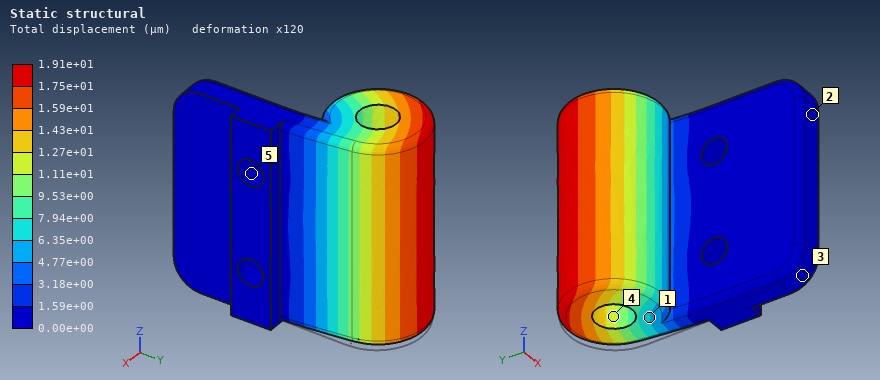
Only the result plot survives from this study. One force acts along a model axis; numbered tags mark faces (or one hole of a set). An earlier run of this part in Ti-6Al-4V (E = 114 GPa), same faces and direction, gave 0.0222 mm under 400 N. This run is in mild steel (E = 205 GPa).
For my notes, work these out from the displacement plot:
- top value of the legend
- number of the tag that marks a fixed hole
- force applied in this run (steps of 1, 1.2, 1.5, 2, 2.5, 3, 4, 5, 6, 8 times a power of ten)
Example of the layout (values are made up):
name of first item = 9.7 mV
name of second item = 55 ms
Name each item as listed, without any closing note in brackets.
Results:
top value of the legend = 1.91e+01 µm
number of the tag that marks a fixed hole = 5
force applied in this run = 600 N
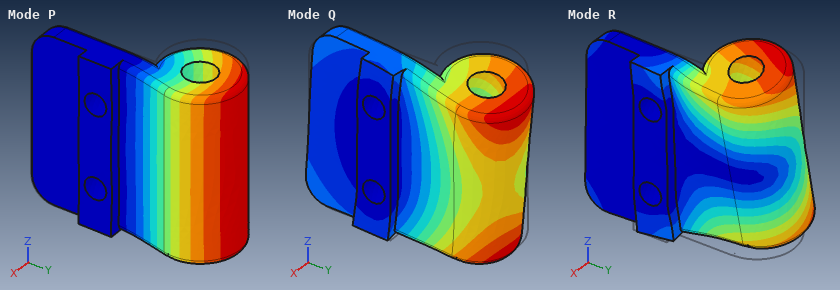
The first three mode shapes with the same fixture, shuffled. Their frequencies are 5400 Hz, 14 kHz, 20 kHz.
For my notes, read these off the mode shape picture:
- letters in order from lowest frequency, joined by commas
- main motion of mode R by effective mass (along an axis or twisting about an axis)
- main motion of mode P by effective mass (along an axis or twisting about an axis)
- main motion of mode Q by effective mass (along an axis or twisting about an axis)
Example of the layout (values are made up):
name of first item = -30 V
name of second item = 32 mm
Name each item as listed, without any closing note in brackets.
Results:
letters in order from lowest frequency, joined by commas = P, R, Q
main motion of mode R by effective mass = along Z
main motion of mode P by effective mass = along X
main motion of mode Q by effective mass = along Z
